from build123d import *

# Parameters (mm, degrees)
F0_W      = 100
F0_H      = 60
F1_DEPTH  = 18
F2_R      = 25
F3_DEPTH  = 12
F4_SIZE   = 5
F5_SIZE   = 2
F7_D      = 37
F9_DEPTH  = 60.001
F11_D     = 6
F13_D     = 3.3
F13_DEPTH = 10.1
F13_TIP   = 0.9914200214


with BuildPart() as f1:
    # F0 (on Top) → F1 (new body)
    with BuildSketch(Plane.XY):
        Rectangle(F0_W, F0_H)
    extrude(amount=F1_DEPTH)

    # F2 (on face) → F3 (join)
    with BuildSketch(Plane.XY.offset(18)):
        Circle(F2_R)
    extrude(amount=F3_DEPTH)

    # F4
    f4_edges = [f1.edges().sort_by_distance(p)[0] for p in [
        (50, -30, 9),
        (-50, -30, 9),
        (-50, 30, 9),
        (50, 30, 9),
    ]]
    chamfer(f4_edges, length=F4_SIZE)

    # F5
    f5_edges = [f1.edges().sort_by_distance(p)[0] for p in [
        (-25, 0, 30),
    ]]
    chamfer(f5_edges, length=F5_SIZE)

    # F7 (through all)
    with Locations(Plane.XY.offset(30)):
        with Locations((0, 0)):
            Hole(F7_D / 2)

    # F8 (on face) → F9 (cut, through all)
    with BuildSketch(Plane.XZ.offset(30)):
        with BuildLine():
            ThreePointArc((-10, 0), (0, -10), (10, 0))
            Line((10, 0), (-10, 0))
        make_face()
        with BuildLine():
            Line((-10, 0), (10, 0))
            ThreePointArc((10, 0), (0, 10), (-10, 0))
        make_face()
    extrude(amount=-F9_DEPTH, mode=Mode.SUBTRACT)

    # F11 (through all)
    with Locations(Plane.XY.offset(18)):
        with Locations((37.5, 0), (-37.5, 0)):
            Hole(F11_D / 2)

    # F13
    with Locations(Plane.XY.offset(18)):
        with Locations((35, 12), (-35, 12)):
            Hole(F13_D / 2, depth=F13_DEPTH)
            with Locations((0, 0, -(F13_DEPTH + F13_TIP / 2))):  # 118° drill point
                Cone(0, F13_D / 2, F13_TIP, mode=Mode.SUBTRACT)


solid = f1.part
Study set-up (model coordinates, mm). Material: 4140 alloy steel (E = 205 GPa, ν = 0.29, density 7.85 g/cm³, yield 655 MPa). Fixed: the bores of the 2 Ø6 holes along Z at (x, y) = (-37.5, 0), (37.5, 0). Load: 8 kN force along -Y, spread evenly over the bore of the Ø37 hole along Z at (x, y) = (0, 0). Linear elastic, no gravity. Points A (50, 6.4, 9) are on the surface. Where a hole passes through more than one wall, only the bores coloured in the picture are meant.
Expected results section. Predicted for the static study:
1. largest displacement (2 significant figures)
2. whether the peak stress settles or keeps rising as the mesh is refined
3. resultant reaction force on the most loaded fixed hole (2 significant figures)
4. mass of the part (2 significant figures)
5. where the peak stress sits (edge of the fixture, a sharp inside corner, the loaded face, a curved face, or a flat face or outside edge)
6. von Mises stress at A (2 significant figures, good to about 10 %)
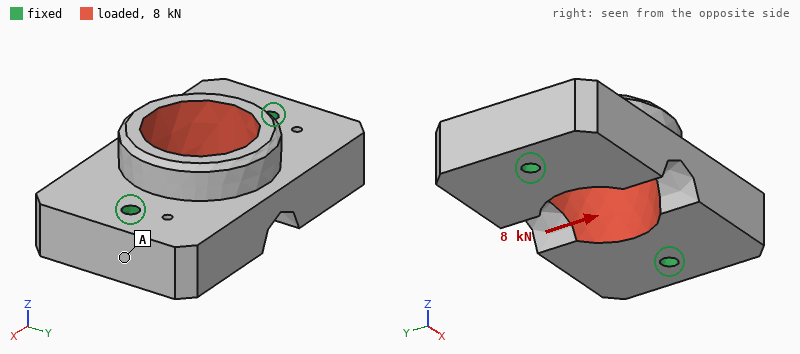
9.1 µm
keeps rising
4.0 kN
730 g
edge of the fixture
6.2 MPa
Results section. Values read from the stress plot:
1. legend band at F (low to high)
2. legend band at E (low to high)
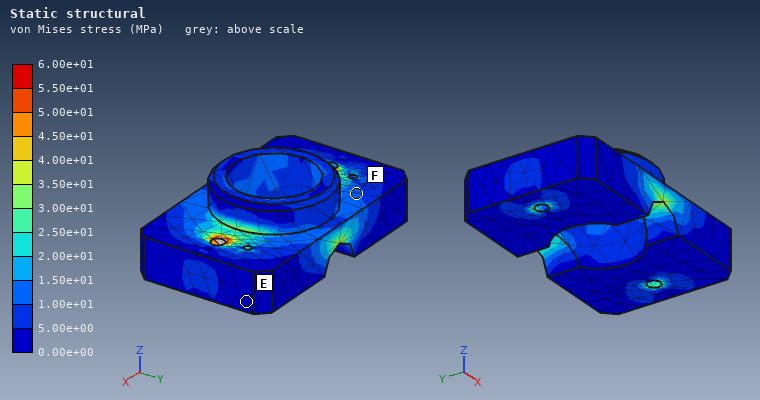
1.00e+01 to 1.50e+01 MPa
0.00e+00 to 5.00e+00 MPa
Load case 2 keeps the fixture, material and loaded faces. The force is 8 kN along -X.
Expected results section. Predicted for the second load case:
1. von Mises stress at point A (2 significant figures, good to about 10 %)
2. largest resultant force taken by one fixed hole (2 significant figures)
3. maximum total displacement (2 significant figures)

5.3 MPa
4.1 kN
2.6 µm
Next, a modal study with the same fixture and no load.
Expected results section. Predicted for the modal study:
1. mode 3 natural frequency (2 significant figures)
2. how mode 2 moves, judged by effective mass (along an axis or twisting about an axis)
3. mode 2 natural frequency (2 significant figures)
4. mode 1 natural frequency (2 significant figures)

10 kHz
along Z
9000 Hz
7200 Hz
